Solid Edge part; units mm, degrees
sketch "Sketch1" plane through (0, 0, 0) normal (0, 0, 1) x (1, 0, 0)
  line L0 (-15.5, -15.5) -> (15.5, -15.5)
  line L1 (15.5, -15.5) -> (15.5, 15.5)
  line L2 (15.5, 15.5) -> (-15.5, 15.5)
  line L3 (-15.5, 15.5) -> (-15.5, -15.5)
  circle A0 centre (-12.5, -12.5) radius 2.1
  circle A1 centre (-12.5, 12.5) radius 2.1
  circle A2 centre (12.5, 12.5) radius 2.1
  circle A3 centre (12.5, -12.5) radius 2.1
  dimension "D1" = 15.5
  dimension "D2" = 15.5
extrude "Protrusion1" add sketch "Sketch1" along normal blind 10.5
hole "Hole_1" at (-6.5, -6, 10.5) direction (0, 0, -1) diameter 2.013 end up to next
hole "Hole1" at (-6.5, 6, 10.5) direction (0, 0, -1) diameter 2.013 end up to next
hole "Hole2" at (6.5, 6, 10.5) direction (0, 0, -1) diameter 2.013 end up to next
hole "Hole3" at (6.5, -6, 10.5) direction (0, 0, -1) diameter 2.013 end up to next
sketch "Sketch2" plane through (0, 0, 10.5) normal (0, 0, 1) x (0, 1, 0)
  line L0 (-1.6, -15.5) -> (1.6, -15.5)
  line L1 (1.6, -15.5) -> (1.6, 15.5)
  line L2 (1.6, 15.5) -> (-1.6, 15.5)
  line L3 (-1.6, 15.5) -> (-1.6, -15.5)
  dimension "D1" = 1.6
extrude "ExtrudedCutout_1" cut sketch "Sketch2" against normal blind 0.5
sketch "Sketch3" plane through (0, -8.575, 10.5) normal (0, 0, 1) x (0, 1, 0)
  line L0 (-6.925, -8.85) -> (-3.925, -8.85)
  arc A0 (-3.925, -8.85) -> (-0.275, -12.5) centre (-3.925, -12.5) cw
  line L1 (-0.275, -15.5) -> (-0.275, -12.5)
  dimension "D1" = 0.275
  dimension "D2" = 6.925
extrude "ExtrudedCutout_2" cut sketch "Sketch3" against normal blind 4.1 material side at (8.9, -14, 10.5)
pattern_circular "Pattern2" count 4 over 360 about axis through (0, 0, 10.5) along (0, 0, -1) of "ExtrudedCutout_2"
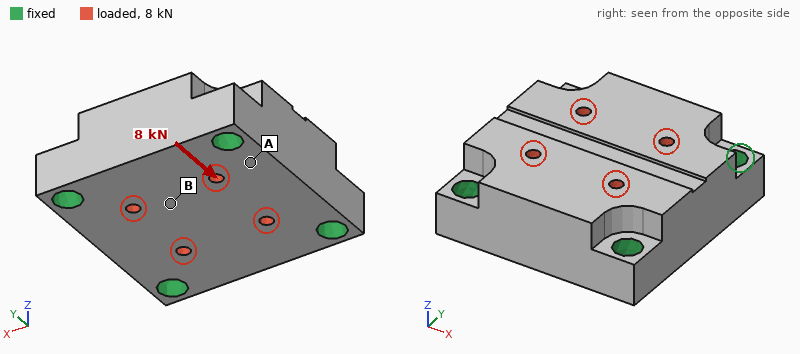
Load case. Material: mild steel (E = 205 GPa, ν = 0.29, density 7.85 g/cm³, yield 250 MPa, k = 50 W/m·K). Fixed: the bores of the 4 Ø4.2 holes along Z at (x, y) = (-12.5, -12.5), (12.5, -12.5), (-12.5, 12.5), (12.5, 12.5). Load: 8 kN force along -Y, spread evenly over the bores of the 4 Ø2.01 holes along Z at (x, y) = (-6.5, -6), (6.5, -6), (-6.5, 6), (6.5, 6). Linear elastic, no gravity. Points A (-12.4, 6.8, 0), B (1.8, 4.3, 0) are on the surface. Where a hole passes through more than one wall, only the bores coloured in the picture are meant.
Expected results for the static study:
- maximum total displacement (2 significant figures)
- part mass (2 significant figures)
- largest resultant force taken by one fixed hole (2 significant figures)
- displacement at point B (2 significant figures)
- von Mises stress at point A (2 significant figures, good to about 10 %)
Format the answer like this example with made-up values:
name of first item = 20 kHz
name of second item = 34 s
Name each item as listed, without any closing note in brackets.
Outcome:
maximum total displacement = 2.1 µm
part mass = 70 g
largest resultant force taken by one fixed hole = 2.1 kN
displacement at point B = 1.6 µm
von Mises stress at point A = 21 MPa
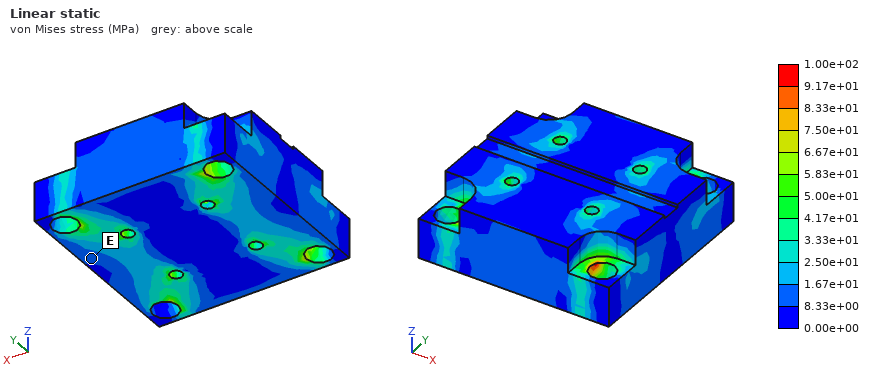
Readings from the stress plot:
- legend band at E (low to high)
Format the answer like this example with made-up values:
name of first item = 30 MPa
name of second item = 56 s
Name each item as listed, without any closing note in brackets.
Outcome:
legend band at E = 8.33e+00 to 1.67e+01 MPa
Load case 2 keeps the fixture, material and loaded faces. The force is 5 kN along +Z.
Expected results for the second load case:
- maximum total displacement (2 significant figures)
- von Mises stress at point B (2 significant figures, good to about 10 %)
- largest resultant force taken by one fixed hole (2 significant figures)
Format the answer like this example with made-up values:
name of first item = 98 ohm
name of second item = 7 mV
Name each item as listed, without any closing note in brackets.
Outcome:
maximum total displacement = 2.7 µm
von Mises stress at point B = 16 MPa
largest resultant force taken by one fixed hole = 1.3 kN
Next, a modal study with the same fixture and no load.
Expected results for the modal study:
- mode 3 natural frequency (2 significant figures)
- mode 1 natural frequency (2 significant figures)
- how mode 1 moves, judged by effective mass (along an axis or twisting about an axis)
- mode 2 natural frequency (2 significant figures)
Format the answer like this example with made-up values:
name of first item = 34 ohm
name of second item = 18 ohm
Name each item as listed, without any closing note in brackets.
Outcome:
mode 3 natural frequency = 46 kHz
mode 1 natural frequency = 34 kHz
how mode 1 moves, judged by effective mass = along Z
mode 2 natural frequency = 46 kHz
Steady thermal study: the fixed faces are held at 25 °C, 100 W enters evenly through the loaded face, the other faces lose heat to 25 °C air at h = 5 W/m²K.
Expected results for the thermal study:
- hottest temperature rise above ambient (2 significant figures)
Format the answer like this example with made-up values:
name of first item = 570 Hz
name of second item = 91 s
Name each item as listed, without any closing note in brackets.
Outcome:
hottest temperature rise above ambient = 51 K
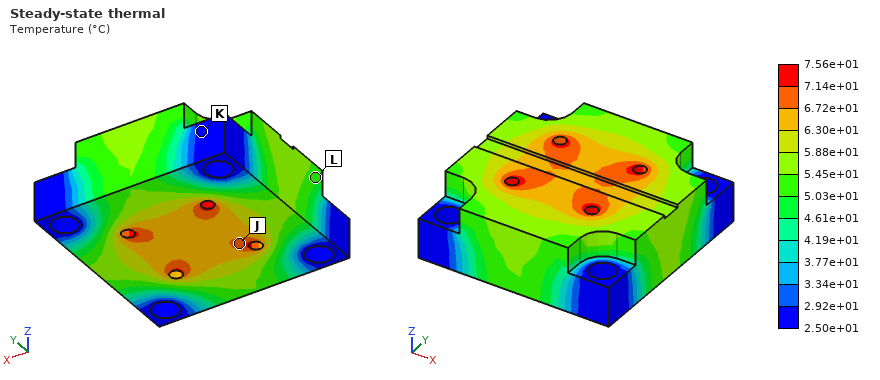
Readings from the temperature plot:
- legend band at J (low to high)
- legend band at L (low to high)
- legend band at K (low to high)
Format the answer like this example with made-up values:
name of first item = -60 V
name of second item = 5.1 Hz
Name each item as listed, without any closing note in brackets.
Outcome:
legend band at J = 6.72e+01 to 7.14e+01 °C
legend band at L = 5.03e+01 to 5.45e+01 °C
legend band at K = 2.50e+01 to 2.92e+01 °C
